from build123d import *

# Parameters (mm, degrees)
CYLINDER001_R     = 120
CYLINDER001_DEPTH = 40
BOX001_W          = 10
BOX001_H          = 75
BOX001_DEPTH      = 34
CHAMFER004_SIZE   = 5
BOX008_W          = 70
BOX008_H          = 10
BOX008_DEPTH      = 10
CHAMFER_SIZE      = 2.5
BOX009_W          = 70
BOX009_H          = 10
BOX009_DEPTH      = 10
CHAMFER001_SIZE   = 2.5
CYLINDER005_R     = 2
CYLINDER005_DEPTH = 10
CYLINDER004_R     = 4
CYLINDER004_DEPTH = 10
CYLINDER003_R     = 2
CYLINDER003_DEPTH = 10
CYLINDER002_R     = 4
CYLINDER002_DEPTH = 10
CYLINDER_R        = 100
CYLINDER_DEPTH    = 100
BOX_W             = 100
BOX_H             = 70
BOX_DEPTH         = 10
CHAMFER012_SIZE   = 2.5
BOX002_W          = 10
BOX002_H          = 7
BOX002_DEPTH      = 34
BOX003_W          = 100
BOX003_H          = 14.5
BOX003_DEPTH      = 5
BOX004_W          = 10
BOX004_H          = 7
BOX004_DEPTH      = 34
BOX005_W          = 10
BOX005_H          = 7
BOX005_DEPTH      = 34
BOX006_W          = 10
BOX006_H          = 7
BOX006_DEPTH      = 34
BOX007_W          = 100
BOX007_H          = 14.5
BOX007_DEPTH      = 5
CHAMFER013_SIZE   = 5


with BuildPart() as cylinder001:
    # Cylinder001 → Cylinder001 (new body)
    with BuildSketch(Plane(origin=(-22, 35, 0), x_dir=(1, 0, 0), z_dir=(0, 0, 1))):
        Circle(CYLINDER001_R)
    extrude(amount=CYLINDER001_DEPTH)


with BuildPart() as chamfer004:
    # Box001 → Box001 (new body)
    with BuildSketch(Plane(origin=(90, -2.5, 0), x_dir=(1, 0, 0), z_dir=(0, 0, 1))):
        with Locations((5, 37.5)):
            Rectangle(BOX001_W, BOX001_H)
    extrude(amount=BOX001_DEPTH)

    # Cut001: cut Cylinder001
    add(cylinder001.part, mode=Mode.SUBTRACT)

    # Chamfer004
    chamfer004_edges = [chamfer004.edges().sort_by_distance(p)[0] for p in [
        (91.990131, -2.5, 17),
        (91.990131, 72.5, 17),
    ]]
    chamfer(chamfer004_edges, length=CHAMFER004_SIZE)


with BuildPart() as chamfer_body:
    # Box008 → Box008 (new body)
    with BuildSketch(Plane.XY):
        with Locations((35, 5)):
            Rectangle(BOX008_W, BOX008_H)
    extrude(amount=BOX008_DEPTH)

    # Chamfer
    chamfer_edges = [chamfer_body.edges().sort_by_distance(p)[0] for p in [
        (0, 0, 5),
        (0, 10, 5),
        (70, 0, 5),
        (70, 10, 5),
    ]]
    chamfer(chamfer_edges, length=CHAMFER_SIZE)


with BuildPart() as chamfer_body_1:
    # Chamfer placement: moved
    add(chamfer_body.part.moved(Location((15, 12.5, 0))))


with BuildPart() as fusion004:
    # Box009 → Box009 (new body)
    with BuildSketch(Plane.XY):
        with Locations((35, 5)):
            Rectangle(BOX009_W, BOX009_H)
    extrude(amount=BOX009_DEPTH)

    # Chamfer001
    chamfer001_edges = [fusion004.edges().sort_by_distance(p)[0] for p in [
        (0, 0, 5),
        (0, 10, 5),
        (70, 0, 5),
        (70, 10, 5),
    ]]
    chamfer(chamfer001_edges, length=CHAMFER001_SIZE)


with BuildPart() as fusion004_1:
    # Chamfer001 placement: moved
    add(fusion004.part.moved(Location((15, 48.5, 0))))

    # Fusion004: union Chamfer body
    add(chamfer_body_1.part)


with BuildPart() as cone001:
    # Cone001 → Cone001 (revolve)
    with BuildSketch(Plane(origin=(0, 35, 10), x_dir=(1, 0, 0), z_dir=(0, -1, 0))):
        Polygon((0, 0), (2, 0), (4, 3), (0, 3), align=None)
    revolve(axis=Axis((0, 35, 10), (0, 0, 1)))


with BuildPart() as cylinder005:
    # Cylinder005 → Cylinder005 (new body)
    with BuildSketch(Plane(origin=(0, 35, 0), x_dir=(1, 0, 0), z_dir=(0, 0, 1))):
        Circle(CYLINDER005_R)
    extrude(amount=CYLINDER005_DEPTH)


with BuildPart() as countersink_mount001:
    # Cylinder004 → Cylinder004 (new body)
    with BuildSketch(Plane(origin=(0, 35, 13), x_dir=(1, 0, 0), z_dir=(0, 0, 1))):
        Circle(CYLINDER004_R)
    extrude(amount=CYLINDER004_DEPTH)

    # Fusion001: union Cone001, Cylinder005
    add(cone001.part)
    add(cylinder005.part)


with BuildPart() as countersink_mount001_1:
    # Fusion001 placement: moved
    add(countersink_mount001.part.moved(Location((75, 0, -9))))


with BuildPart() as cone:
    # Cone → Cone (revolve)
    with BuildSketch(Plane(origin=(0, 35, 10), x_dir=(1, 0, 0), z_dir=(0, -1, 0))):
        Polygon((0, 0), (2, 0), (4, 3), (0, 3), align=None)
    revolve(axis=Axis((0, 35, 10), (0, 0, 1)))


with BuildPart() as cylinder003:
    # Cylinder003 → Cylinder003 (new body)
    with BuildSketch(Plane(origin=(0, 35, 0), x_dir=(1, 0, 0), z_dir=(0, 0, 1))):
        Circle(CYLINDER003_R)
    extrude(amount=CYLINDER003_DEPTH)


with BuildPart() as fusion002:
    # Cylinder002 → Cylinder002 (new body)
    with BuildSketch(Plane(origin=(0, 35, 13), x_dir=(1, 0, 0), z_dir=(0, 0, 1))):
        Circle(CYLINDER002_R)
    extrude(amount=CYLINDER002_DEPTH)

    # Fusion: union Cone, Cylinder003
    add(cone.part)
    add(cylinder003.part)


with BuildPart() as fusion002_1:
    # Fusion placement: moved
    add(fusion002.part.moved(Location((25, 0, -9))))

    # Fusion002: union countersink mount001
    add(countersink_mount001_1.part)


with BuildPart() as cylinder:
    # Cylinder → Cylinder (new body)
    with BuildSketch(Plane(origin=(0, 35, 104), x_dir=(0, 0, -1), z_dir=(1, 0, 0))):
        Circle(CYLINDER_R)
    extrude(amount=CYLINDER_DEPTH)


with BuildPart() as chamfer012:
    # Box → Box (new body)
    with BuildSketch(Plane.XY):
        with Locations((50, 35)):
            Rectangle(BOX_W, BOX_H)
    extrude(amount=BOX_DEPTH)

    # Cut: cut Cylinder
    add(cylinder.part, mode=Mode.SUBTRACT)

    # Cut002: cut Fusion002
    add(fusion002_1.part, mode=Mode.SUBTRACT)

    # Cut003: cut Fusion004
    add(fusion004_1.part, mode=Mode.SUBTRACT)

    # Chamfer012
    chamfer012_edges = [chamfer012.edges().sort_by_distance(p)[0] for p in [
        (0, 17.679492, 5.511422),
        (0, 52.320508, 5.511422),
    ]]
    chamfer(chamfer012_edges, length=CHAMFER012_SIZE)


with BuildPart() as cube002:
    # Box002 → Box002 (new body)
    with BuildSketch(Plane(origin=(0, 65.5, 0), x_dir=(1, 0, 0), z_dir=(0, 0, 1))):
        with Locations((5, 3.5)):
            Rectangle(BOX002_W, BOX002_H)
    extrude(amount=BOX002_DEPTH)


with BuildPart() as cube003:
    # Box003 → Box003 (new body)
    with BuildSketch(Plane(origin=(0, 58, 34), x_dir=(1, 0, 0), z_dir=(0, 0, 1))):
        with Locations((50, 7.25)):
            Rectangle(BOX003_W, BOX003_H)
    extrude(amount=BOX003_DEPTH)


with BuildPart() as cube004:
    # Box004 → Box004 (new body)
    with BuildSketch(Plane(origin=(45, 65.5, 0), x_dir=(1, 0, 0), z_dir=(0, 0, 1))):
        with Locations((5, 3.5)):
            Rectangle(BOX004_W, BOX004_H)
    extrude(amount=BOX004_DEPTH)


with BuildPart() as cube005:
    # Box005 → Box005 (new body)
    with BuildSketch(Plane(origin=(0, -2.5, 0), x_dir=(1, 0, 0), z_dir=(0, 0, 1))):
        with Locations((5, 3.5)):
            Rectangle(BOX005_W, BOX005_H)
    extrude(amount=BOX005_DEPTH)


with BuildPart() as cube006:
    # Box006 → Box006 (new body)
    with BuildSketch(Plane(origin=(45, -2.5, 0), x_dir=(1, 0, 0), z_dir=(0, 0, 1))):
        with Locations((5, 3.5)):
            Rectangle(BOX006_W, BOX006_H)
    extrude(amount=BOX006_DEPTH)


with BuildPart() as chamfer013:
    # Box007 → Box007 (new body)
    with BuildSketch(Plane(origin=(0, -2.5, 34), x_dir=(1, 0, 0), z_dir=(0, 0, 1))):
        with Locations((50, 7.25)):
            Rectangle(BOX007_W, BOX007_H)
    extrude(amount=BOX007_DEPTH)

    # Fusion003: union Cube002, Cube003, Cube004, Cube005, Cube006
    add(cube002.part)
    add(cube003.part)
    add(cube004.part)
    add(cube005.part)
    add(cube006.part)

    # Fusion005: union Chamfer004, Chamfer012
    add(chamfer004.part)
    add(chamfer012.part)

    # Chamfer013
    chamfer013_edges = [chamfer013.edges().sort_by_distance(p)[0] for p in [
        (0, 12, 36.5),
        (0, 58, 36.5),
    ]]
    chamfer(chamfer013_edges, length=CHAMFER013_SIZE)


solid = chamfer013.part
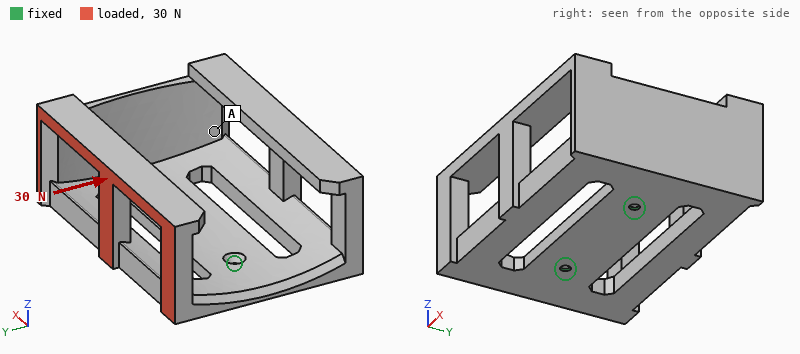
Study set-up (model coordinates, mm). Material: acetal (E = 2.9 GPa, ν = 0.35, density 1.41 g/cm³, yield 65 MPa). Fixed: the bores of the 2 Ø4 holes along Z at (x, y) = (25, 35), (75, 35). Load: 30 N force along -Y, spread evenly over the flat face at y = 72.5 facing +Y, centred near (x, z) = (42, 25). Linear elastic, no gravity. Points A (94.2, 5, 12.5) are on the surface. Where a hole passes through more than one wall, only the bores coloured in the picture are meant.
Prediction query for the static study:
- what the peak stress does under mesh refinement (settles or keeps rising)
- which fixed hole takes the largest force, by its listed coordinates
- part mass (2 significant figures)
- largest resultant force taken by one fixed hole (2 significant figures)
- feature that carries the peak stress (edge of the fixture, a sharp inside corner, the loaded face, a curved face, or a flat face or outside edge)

keeps rising
(25, 35)
90 g
20 N
edge of the fixture
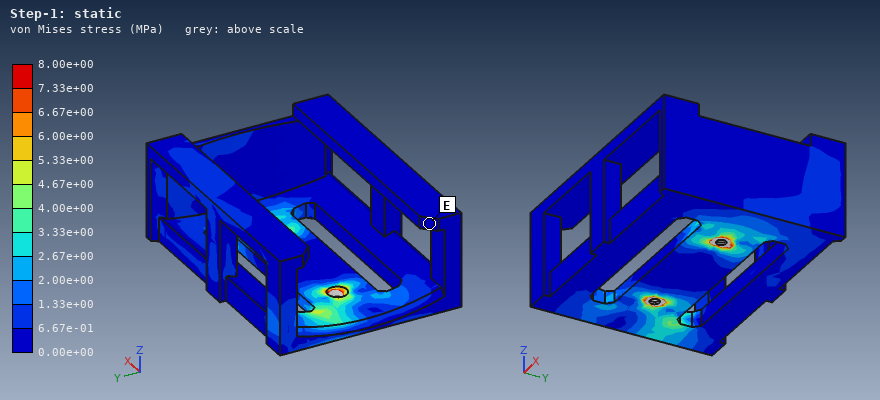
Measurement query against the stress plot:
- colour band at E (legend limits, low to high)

0.00e+00 to 6.67e-01 MPa
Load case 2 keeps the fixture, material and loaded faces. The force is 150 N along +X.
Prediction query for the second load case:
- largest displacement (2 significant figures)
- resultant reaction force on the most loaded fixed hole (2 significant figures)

0.95 mm
150 N
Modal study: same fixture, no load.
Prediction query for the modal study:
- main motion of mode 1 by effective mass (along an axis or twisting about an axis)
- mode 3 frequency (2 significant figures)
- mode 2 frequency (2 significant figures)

along Y
350 Hz
270 Hz
